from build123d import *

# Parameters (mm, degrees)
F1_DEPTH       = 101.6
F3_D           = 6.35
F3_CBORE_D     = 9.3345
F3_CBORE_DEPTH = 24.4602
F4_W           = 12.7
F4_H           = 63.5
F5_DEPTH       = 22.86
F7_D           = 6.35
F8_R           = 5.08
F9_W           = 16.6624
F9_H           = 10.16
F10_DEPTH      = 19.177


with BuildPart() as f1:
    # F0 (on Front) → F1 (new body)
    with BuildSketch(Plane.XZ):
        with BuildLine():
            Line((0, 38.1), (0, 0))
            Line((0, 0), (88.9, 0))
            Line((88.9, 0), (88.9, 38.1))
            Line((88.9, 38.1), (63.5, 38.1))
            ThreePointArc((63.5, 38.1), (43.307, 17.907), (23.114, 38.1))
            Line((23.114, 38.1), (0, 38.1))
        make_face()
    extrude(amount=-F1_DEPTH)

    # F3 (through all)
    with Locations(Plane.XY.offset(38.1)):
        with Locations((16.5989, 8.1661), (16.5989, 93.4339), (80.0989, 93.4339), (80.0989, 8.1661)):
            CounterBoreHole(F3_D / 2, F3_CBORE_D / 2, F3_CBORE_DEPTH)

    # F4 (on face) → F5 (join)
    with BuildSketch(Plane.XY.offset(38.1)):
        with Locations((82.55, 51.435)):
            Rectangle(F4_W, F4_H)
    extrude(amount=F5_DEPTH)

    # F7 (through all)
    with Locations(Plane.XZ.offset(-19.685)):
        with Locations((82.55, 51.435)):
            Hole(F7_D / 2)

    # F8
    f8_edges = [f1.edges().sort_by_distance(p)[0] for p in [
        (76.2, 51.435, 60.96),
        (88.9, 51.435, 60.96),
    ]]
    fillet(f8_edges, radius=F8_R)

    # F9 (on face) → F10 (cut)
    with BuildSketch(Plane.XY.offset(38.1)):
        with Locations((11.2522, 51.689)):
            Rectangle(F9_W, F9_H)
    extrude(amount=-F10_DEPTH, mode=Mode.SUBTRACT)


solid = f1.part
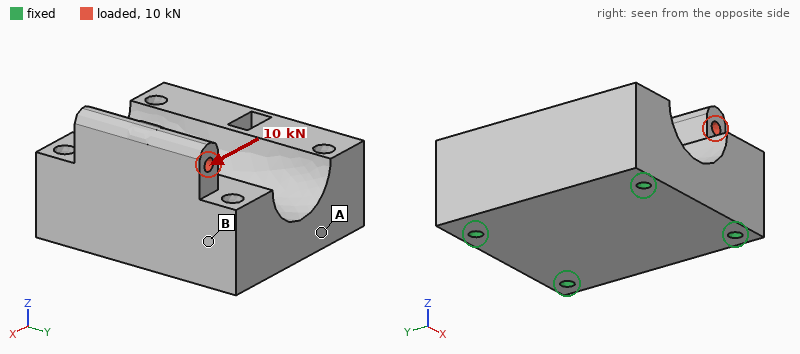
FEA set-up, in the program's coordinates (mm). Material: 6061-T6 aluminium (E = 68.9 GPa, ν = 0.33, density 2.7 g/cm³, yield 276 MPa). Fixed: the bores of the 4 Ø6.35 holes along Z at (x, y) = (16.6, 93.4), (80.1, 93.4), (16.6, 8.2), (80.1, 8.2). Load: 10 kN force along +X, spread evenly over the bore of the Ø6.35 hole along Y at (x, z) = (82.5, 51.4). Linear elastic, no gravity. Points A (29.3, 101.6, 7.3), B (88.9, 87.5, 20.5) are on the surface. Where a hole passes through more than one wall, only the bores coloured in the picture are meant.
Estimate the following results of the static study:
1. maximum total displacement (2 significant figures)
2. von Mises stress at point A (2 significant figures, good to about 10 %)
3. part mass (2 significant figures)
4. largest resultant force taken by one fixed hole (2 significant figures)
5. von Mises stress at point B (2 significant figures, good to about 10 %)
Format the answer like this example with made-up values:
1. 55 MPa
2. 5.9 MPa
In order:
1. 0.13 mm
2. 14 MPa
3. 760 g
4. 5.0 kN
5. 31 MPa
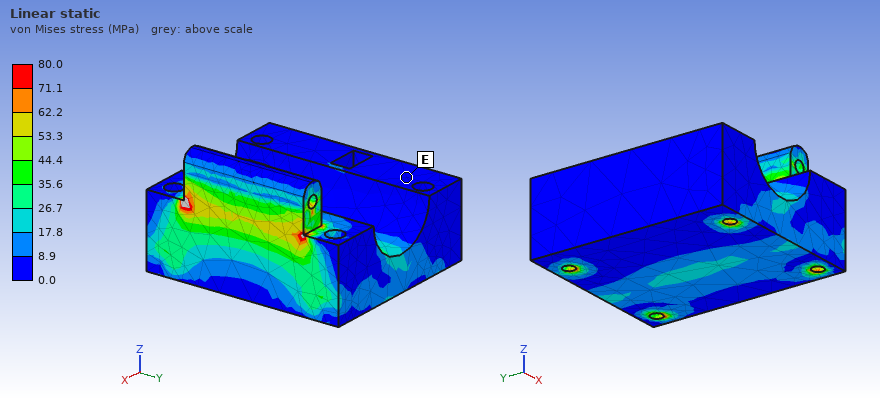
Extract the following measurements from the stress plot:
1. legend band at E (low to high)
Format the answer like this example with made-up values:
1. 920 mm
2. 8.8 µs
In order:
1. 0.0 to 8.9 MPa
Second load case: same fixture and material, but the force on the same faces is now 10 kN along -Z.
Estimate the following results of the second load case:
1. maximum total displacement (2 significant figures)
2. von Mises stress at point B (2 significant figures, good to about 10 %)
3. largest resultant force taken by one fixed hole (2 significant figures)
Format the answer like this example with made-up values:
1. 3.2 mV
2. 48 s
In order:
1. 25 µm
2. 22 MPa
3. 5.7 kN
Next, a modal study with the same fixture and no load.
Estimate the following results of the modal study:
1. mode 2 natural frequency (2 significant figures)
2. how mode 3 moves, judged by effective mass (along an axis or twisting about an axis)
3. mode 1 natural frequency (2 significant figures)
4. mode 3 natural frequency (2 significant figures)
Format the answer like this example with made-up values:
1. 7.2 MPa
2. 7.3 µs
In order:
1. 8500 Hz
2. along Z
3. 6900 Hz
4. 8900 Hz
